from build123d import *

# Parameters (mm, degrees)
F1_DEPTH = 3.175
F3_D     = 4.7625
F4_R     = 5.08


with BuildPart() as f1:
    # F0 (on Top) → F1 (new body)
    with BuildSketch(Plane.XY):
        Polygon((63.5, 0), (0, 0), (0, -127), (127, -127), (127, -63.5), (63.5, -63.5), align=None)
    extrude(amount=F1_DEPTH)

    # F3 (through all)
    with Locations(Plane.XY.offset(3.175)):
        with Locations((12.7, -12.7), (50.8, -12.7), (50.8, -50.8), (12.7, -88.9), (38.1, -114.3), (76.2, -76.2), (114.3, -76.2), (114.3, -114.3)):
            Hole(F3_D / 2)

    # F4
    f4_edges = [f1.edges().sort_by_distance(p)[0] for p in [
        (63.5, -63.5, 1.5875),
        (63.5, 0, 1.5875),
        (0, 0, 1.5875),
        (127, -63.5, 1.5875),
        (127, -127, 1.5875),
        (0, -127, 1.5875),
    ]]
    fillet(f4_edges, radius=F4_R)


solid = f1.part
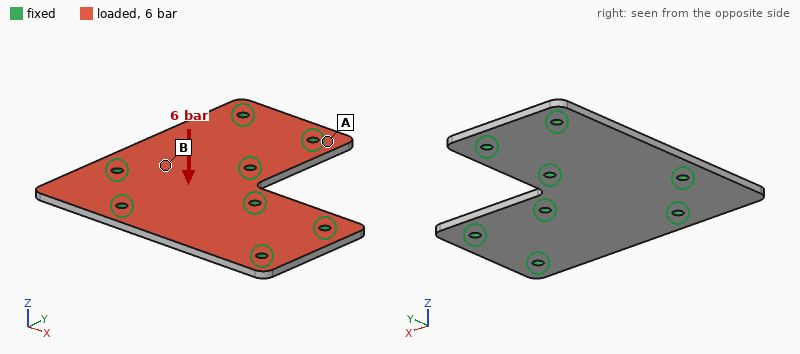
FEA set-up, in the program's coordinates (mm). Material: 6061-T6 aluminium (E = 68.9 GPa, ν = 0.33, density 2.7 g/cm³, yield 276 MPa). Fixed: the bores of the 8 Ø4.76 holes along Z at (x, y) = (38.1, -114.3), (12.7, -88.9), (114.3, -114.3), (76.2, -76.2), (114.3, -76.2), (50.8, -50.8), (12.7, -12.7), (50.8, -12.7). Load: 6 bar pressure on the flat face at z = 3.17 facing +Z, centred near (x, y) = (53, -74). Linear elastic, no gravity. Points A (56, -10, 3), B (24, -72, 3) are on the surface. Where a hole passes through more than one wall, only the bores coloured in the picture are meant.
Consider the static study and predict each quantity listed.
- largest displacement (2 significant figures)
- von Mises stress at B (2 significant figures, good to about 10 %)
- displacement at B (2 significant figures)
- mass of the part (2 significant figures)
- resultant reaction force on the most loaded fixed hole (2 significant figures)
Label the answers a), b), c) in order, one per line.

a) 0.27 mm
b) 51 MPa
c) 0.094 mm
d) 100 g
e) 1.2 kN
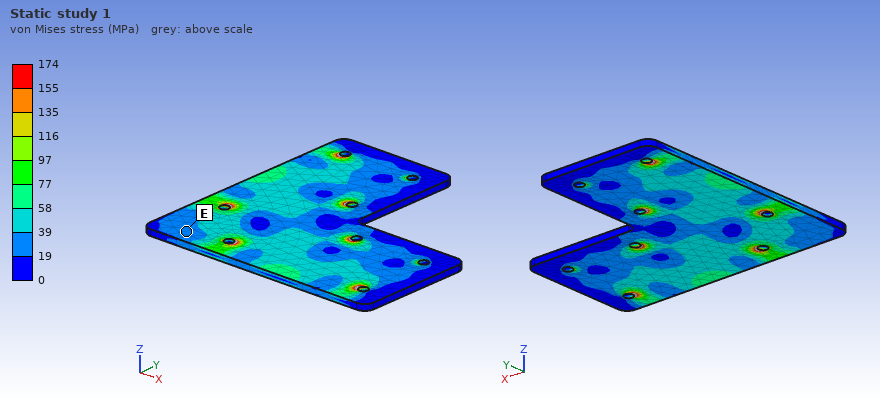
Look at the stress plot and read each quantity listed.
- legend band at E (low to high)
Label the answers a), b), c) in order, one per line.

a) 19 to 39 MPa
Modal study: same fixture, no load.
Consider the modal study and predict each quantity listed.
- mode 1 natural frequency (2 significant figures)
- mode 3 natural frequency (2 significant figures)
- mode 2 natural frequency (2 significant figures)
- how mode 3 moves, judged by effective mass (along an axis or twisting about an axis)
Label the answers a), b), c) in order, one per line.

a) 3300 Hz
b) 3600 Hz
c) 3300 Hz
d) along Z
